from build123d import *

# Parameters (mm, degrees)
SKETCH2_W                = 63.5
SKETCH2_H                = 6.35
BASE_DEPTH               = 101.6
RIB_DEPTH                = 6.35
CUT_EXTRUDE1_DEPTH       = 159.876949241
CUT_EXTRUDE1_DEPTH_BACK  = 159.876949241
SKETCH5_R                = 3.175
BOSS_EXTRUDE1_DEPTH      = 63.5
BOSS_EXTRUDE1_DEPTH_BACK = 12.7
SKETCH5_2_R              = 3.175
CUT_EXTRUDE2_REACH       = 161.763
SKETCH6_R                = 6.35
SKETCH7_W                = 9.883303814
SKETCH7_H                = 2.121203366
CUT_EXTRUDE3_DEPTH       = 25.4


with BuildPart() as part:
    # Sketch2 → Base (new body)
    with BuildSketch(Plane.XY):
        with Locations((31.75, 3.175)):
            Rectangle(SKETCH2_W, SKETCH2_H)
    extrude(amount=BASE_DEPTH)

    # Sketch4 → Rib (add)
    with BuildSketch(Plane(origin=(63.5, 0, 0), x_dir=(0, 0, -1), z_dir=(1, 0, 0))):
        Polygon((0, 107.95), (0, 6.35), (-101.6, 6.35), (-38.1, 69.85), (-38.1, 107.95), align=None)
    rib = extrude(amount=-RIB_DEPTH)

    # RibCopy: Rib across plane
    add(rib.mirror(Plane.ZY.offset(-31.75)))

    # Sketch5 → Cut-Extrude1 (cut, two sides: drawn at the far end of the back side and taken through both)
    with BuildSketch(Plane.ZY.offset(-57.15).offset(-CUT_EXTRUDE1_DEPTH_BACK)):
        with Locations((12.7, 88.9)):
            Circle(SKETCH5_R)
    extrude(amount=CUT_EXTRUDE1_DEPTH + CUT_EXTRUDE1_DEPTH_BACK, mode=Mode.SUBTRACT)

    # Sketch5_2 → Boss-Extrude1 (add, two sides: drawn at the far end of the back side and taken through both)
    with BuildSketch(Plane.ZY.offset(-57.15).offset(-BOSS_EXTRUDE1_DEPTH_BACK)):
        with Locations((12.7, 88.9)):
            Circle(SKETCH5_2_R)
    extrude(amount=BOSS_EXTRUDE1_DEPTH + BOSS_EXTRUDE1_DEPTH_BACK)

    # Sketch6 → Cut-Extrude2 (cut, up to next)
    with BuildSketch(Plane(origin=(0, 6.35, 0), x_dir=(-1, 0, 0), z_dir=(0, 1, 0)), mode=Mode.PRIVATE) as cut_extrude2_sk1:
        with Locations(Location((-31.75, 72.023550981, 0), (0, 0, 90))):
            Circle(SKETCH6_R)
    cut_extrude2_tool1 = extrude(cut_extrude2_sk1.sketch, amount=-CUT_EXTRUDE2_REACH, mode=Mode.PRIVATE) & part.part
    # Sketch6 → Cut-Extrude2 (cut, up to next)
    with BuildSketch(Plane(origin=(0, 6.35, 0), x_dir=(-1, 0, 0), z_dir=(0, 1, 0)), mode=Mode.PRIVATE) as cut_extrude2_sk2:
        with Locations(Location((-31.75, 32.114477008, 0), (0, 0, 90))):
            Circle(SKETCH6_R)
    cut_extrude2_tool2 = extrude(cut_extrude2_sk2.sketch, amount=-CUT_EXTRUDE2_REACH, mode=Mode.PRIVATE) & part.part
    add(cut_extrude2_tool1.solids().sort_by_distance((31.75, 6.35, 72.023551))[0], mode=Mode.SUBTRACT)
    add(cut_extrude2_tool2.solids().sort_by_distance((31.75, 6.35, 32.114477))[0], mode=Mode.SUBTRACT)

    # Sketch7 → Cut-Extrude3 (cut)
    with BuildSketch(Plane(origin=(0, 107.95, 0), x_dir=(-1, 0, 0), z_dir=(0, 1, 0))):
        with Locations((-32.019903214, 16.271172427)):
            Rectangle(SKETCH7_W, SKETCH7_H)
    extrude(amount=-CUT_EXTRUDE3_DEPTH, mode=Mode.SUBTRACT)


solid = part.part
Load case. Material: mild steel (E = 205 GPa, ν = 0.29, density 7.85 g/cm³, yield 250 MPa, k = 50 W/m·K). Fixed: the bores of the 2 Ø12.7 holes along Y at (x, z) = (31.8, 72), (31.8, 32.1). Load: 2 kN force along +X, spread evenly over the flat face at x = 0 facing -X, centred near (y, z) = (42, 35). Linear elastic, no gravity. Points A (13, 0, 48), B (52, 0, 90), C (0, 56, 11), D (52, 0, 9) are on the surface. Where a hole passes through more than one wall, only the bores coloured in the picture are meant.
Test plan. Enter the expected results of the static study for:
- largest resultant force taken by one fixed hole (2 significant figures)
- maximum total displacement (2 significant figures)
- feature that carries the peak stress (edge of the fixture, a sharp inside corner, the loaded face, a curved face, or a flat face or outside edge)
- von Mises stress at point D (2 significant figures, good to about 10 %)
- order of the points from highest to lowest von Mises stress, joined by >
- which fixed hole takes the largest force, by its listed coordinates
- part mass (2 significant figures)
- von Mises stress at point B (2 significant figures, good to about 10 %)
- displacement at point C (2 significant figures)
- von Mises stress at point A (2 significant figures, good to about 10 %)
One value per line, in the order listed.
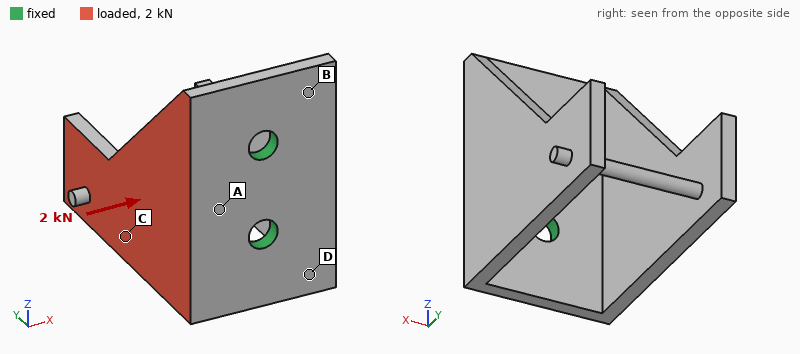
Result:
1.7 kN
0.45 mm
a curved face
44 MPa
A > D > B > C
(31.8, 32.1)
910 g
26 MPa
0.23 mm
64 MPa
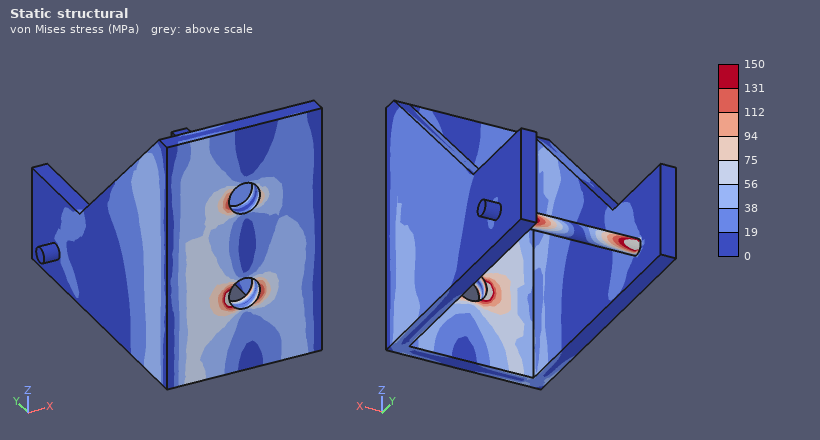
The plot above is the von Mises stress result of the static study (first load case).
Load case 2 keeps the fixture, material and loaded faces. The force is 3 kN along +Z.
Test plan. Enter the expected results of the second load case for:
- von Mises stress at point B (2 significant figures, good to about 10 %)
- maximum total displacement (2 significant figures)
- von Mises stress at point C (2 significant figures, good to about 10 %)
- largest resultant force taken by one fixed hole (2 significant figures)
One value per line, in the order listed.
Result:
15 MPa
0.15 mm
15 MPa
3.2 kN
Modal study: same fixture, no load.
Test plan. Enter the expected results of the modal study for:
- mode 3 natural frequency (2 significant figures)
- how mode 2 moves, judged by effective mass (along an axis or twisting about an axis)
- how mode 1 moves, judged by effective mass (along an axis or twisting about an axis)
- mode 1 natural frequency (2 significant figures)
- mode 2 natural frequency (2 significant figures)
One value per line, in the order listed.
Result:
1500 Hz
along Z
along X
510 Hz
1400 Hz
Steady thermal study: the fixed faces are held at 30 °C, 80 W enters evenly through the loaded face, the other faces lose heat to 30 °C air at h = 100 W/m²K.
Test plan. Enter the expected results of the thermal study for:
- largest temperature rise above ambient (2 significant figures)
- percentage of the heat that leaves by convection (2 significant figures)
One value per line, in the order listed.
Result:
63 K
67 %
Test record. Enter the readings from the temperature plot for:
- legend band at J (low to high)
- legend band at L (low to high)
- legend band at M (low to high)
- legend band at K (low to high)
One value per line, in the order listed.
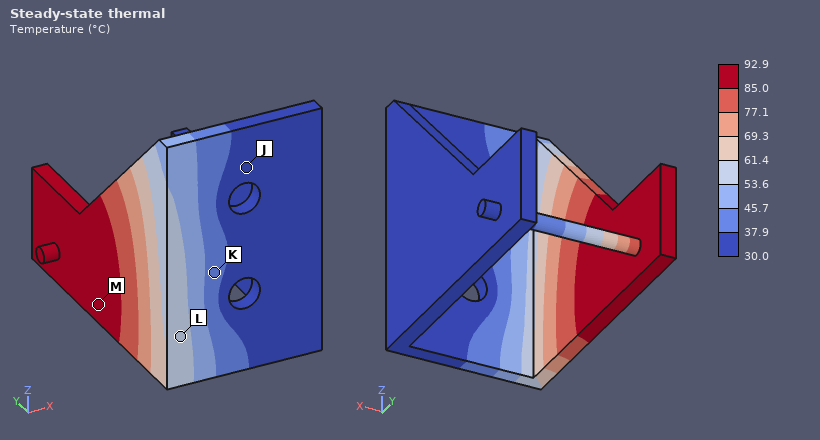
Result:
30.0 to 37.9 °C
53.6 to 61.4 °C
85.0 to 92.9 °C
37.9 to 45.7 °C
